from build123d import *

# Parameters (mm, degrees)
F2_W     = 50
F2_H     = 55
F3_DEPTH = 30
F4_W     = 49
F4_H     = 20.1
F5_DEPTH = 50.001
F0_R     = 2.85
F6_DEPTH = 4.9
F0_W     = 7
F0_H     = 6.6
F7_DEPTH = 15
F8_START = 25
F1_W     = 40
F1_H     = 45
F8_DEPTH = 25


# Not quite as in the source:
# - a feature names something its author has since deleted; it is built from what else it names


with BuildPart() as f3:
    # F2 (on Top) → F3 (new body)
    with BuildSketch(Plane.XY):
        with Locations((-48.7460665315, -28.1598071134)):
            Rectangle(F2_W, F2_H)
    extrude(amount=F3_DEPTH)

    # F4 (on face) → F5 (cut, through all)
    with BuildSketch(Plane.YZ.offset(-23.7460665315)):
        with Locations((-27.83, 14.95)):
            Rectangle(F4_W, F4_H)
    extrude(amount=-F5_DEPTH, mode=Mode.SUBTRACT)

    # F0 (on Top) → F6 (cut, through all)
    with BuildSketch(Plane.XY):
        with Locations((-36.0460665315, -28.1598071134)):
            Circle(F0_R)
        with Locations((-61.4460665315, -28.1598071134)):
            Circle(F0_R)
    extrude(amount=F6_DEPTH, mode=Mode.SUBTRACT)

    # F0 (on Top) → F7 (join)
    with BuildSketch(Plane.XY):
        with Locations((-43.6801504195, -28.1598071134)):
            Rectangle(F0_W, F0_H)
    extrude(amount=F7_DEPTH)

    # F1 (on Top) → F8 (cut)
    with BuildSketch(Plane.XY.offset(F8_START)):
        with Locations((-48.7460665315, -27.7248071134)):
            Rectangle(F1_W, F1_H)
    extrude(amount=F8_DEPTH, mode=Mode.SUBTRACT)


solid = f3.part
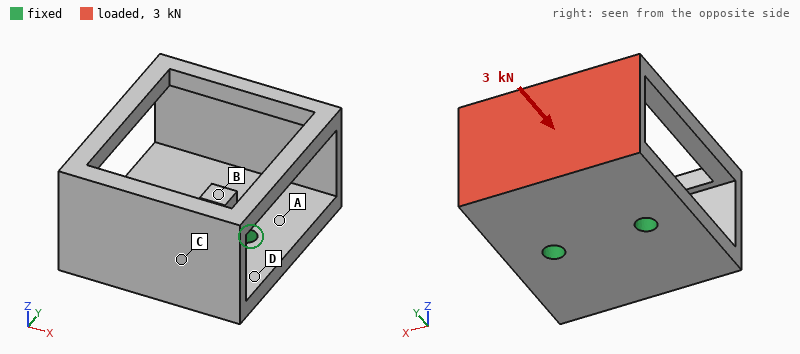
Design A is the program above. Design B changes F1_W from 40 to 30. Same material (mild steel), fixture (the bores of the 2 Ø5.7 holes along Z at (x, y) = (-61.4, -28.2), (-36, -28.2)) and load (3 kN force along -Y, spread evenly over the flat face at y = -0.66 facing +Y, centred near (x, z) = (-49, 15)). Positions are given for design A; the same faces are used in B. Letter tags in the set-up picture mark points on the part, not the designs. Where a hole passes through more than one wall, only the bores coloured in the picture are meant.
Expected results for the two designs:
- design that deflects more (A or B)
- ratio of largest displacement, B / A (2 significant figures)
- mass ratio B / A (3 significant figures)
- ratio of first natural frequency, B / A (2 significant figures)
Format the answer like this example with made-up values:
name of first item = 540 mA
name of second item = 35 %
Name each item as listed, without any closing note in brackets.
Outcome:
design that deflects more = A
ratio of largest displacement, B / A = 0.81
mass ratio B / A = 1.09
ratio of first natural frequency, B / A = 0.93
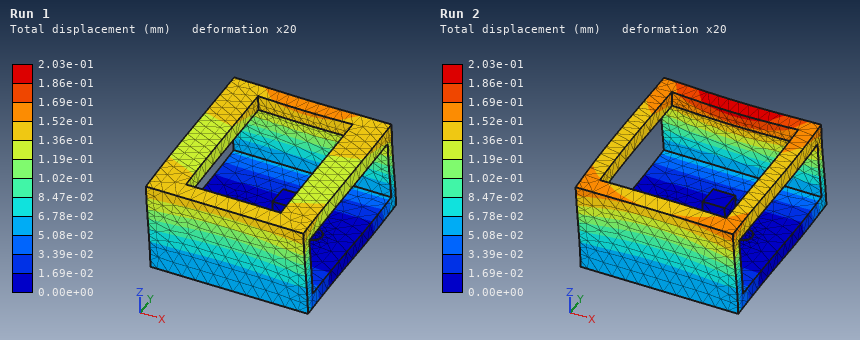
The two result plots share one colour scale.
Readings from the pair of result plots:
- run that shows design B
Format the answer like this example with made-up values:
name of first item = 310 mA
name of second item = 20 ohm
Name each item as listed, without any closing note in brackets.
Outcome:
run that shows design B = Run 1
